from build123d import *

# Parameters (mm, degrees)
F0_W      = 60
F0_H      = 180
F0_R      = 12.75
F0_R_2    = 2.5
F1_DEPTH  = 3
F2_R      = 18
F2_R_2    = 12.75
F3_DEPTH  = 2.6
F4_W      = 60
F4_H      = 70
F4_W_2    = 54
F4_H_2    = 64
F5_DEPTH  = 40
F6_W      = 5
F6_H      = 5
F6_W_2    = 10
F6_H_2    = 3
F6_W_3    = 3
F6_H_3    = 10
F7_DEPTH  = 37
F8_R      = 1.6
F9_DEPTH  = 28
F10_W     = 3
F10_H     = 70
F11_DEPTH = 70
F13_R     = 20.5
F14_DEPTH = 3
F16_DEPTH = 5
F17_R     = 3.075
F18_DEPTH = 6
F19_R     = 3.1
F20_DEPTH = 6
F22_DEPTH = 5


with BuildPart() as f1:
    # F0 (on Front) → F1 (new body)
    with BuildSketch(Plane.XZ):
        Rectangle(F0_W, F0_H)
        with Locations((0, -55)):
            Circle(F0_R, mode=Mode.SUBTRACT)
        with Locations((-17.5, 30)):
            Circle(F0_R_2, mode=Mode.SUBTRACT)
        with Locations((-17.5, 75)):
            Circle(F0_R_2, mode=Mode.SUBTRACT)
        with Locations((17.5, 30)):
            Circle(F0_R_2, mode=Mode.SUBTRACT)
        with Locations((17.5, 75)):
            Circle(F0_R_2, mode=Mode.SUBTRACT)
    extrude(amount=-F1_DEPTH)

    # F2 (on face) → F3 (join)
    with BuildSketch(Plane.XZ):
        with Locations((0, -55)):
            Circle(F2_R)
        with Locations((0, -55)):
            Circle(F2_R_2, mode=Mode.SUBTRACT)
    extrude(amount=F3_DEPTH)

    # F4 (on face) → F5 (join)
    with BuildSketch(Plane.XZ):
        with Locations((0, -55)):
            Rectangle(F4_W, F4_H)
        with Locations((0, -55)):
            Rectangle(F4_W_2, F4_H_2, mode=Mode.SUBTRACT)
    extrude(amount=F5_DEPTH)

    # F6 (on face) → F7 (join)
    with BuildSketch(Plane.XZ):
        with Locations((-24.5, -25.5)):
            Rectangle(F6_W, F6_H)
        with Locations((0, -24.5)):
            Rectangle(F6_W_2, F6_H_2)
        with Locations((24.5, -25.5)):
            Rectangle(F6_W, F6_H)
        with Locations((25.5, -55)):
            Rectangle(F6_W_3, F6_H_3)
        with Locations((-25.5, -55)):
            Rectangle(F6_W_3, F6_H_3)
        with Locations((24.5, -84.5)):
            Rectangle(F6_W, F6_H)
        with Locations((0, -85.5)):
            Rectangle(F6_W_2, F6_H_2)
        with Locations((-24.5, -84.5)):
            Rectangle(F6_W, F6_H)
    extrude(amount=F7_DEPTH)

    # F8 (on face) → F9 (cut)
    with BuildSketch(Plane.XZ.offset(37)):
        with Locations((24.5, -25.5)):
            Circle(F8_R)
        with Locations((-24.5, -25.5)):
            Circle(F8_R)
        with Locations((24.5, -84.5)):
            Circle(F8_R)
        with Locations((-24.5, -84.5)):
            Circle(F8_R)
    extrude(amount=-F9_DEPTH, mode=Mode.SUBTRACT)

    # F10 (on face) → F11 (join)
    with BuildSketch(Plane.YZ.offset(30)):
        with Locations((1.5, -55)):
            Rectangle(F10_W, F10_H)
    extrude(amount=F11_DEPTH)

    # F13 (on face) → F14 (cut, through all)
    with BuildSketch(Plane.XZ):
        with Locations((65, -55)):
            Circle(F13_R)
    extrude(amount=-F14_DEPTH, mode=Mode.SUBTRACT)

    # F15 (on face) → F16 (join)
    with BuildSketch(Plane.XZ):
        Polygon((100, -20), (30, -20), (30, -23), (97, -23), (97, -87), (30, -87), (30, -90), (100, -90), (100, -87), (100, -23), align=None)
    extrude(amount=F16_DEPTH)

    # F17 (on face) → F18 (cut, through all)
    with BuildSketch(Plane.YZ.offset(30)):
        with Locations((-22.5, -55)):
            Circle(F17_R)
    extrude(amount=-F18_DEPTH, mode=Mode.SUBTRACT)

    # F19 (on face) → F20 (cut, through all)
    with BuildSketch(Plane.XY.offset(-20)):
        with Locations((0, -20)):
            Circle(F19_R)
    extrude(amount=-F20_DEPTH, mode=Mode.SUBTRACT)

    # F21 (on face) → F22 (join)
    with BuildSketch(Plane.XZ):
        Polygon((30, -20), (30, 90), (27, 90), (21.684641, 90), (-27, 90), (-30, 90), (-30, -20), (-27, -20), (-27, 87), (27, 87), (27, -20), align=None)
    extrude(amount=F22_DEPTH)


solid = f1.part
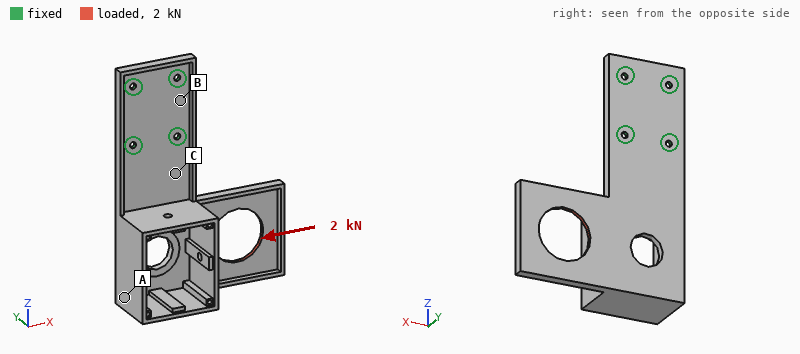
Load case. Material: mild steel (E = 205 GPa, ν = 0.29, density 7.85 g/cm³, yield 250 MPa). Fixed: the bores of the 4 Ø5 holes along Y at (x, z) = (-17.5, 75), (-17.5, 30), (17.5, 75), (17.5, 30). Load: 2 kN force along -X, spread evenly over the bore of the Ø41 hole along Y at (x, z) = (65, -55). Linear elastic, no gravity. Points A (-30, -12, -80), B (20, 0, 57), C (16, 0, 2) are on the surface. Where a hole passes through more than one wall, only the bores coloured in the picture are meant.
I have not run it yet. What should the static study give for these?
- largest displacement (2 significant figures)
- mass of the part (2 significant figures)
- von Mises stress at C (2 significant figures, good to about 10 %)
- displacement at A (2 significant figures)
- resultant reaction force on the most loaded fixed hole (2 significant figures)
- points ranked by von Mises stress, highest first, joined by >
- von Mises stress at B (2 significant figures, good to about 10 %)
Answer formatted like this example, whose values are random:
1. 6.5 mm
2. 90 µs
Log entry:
1. 99 µm
2. 680 g
3. 32 MPa
4. 68 µm
5. 3.5 kN
6. C > B > A
7. 13 MPa
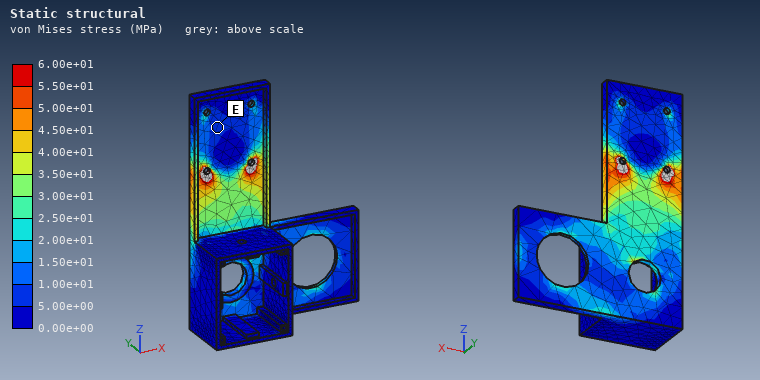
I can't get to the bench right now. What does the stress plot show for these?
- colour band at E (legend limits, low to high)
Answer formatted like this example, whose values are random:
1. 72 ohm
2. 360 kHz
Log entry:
1. 5.00e+00 to 1.00e+01 MPa
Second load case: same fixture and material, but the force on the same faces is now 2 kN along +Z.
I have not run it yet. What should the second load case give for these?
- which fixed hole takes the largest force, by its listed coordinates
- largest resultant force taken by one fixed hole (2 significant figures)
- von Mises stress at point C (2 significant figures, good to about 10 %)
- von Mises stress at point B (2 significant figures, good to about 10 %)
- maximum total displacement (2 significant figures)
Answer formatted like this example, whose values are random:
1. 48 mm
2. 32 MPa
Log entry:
1. (17.5, 30)
2. 3.3 kN
3. 36 MPa
4. 11 MPa
5. 0.13 mm
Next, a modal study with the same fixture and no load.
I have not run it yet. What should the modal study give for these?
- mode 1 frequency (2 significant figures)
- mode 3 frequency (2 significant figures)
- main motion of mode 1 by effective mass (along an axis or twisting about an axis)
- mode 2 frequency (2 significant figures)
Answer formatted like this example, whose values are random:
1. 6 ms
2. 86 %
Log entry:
1. 140 Hz
2. 1000 Hz
3. along Y
4. 310 Hz
